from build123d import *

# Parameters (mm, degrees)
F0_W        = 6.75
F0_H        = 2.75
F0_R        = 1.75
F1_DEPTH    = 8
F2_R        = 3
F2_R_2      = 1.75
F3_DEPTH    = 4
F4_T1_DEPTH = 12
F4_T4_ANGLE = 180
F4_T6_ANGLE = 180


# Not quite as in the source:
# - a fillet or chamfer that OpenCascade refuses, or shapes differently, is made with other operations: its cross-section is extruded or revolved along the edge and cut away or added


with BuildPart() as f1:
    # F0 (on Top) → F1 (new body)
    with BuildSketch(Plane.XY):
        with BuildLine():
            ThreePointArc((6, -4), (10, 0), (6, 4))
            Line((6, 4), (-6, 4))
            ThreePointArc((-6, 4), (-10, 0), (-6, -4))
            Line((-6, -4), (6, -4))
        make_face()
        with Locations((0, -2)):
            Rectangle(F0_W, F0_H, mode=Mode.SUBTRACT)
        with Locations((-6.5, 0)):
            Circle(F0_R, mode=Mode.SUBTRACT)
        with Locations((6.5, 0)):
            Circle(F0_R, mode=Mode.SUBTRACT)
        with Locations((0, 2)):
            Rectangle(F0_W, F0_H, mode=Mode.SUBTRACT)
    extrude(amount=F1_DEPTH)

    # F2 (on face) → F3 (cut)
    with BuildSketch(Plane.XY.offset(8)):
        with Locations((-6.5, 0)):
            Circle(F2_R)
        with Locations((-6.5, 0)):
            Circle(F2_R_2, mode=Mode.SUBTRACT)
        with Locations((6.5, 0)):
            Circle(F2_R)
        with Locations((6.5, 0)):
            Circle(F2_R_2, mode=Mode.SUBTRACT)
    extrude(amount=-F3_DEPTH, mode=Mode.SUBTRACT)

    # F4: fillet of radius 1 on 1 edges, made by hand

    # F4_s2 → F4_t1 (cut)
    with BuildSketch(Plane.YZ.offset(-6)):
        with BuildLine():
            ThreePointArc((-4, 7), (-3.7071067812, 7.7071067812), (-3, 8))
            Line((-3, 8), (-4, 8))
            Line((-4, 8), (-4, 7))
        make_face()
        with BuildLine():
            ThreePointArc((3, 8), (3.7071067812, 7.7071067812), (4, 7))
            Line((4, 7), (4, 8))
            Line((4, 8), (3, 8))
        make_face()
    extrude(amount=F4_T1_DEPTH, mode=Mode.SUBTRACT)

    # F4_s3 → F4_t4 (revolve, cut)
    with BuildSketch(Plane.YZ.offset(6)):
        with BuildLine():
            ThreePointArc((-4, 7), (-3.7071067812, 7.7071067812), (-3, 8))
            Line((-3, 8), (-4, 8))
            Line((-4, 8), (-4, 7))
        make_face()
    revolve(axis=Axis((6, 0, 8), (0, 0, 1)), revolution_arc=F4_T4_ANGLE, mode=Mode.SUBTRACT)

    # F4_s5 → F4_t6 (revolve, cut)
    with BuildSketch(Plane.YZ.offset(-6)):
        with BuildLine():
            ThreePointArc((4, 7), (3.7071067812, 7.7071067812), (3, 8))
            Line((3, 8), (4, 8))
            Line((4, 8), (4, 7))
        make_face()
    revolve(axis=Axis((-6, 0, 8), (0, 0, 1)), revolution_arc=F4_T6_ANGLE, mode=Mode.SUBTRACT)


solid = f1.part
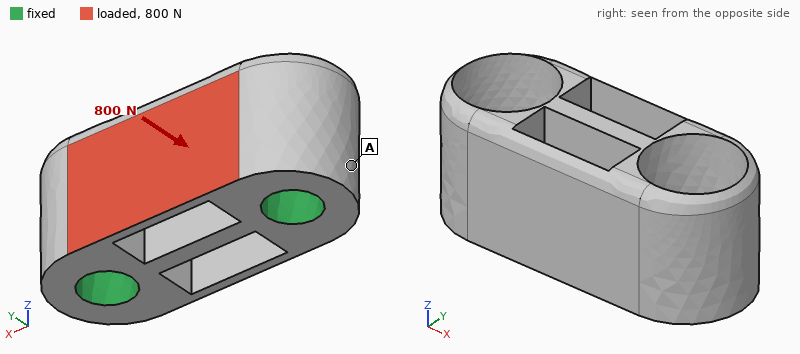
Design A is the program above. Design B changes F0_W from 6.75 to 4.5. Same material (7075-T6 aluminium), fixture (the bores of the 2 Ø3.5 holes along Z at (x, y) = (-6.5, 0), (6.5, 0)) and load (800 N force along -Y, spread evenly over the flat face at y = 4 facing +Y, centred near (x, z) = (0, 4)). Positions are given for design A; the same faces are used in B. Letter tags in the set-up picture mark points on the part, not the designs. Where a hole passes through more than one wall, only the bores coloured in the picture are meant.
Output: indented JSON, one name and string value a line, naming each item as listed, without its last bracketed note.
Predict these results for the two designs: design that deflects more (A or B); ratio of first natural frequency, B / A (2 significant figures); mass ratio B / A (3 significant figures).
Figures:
{
  "design that deflects more": "A",
  "ratio of first natural frequency, B / A": "1.2",
  "mass ratio B / A": "1.18"
}
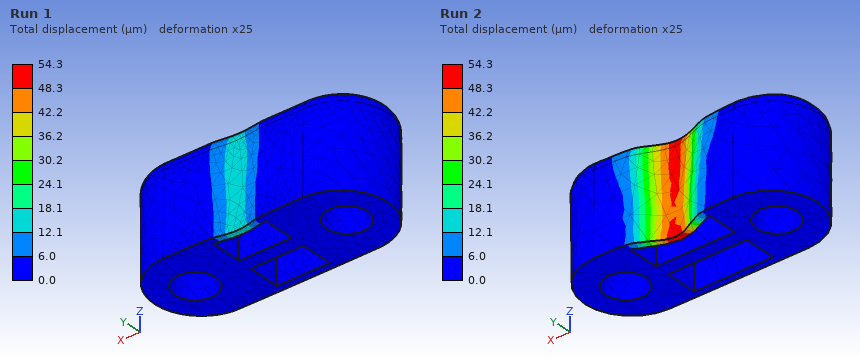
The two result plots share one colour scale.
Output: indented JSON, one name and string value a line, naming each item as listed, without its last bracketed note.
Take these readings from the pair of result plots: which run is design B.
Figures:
{
  "which run is design B": "Run 1"
}
